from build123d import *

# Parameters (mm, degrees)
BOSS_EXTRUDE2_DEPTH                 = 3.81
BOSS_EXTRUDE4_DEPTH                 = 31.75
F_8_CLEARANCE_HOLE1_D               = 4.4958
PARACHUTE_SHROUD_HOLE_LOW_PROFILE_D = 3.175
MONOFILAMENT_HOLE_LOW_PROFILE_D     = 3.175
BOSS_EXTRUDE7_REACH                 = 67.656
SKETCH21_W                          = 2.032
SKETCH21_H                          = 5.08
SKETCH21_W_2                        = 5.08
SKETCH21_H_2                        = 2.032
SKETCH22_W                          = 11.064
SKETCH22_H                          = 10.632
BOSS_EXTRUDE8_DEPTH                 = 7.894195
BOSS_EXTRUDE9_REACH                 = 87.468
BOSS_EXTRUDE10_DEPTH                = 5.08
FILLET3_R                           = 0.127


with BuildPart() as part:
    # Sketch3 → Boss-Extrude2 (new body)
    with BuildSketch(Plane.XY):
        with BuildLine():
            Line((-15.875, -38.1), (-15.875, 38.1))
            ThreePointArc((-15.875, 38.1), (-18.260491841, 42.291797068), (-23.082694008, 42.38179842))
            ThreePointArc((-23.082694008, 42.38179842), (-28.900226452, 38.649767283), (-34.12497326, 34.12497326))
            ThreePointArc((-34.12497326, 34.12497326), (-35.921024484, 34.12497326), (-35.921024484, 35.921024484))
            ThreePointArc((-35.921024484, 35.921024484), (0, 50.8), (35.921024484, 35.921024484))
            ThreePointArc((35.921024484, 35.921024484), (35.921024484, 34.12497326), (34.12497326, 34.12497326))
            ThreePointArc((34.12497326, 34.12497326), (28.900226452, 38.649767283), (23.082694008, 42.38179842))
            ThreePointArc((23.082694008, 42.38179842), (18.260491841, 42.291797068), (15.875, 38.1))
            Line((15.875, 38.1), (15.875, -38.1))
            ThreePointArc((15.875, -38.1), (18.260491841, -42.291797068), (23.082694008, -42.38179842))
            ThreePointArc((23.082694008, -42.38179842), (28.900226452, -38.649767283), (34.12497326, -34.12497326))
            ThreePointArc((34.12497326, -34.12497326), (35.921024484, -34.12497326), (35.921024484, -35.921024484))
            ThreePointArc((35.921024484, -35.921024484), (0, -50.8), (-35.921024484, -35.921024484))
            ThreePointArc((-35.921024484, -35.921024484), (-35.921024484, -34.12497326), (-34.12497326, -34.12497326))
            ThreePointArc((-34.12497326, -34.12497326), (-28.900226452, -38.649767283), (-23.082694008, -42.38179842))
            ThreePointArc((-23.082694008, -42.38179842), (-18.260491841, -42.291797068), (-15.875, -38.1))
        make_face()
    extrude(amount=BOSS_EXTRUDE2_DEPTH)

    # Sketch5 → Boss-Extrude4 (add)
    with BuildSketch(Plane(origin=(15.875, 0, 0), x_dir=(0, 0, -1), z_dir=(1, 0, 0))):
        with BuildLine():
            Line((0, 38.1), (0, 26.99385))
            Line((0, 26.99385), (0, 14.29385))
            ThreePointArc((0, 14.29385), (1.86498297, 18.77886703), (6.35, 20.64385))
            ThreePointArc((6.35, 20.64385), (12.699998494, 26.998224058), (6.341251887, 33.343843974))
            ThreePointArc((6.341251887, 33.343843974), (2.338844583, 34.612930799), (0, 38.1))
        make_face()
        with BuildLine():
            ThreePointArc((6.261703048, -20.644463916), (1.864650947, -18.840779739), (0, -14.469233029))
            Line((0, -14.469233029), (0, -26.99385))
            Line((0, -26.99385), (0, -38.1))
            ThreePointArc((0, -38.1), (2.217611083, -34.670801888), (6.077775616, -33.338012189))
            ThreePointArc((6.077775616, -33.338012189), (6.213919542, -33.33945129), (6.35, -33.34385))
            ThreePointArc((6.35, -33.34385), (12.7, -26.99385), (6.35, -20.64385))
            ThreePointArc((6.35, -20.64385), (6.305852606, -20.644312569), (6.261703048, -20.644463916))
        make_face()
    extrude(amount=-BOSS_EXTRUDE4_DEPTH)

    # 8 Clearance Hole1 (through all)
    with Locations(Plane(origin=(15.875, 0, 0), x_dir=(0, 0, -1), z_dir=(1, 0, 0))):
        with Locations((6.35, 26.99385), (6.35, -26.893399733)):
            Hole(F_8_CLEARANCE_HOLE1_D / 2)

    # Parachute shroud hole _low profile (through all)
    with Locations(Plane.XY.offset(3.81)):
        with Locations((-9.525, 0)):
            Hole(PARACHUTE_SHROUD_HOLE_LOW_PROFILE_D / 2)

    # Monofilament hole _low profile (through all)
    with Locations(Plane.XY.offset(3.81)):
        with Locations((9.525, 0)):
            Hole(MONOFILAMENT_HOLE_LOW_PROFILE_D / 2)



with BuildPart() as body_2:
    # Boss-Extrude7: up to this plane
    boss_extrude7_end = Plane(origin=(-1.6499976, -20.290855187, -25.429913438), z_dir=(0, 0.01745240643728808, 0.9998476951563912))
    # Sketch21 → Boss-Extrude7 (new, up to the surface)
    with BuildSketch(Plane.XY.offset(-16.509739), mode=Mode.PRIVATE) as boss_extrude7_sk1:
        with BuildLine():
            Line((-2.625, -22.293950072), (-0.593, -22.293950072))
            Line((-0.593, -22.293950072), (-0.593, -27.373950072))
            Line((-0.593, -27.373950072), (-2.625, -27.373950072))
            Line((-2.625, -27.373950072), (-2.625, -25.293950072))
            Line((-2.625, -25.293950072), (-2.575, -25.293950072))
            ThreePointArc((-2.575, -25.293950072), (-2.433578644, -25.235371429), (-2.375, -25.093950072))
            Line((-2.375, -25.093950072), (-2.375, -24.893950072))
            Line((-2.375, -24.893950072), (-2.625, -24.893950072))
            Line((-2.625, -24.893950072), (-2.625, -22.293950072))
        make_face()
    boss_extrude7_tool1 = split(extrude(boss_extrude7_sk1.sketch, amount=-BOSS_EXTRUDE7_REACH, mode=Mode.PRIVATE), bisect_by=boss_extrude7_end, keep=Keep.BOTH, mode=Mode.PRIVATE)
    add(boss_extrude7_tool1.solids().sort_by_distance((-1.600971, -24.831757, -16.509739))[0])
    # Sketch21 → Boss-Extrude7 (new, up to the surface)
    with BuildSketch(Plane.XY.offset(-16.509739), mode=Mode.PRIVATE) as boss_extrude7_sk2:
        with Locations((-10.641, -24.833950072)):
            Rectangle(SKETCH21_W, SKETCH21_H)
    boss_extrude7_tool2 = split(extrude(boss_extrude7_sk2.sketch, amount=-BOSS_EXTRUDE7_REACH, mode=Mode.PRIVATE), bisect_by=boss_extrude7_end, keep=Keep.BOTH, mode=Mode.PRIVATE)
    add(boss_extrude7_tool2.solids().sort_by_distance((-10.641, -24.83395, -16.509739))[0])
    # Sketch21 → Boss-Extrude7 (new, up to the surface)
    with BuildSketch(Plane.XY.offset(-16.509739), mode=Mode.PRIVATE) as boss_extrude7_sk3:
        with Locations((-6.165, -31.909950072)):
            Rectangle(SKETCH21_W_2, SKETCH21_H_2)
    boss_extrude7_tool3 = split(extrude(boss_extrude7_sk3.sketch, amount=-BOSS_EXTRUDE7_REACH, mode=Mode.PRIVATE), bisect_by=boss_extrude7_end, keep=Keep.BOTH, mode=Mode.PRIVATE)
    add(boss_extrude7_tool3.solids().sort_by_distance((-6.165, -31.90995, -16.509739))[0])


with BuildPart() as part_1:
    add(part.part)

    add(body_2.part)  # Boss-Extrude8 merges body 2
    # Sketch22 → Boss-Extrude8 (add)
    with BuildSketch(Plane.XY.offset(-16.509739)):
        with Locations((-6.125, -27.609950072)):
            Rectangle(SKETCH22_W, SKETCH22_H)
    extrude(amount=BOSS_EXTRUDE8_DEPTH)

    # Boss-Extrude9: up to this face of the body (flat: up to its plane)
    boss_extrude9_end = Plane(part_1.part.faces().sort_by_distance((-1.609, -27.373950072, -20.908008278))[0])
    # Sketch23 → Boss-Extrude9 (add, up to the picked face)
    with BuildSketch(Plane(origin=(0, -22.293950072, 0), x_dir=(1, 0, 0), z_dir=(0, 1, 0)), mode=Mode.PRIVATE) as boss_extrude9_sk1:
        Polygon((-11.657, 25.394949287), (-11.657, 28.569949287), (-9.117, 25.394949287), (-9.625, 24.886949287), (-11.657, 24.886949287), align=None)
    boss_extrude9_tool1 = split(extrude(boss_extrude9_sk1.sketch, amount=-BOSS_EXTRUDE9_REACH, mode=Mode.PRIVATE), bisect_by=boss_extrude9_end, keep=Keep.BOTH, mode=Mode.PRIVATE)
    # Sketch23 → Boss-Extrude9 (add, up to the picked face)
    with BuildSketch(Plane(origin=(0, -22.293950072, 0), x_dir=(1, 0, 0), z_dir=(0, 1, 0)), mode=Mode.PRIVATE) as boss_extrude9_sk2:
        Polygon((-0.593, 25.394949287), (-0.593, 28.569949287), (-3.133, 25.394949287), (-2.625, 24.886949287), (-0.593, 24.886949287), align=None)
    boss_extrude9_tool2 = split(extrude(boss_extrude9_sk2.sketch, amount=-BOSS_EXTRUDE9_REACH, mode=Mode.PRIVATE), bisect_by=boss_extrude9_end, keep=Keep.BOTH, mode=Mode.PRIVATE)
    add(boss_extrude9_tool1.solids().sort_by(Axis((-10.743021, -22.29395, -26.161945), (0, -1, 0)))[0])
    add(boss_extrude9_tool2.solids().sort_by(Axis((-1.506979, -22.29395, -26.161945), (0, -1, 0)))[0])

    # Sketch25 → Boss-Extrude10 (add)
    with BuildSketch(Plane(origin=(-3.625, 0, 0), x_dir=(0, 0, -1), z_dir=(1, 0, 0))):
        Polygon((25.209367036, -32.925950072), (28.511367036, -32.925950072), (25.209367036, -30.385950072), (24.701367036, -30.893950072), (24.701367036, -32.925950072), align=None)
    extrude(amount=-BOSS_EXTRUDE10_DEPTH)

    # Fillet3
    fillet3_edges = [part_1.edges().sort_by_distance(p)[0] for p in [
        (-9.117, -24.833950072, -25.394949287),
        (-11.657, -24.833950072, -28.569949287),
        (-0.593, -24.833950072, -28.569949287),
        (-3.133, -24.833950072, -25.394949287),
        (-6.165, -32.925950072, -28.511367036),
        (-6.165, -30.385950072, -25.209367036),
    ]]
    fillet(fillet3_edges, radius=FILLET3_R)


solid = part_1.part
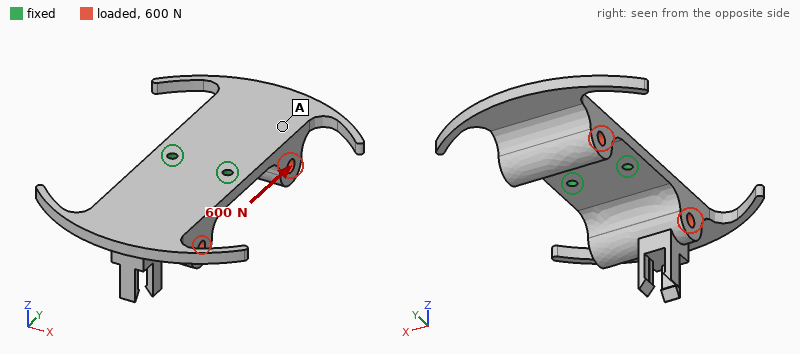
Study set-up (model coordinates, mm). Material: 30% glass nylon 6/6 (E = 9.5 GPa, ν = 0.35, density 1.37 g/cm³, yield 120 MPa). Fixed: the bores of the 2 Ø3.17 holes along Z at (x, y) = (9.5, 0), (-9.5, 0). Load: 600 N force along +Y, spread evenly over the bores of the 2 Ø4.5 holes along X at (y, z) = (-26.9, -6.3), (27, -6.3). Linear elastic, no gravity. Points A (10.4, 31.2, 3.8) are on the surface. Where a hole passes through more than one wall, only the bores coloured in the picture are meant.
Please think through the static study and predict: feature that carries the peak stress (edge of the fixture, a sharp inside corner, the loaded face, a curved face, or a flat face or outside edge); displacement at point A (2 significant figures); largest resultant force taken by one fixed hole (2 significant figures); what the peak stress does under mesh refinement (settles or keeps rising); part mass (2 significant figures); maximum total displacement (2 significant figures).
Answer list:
edge of the fixture
0.75 mm
300 N
keeps rising
32 g
1.4 mm
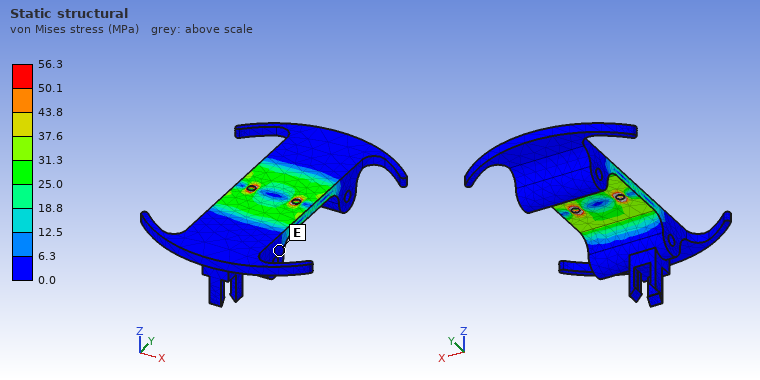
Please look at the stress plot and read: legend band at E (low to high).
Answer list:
0.0 to 6.3 MPa
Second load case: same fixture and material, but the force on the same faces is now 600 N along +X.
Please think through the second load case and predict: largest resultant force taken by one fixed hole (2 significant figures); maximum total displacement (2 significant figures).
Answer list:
370 N
0.32 mm
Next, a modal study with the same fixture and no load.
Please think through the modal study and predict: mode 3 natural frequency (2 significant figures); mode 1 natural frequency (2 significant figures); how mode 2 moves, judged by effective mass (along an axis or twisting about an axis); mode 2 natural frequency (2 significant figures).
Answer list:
1500 Hz
470 Hz
along Z
530 Hz
